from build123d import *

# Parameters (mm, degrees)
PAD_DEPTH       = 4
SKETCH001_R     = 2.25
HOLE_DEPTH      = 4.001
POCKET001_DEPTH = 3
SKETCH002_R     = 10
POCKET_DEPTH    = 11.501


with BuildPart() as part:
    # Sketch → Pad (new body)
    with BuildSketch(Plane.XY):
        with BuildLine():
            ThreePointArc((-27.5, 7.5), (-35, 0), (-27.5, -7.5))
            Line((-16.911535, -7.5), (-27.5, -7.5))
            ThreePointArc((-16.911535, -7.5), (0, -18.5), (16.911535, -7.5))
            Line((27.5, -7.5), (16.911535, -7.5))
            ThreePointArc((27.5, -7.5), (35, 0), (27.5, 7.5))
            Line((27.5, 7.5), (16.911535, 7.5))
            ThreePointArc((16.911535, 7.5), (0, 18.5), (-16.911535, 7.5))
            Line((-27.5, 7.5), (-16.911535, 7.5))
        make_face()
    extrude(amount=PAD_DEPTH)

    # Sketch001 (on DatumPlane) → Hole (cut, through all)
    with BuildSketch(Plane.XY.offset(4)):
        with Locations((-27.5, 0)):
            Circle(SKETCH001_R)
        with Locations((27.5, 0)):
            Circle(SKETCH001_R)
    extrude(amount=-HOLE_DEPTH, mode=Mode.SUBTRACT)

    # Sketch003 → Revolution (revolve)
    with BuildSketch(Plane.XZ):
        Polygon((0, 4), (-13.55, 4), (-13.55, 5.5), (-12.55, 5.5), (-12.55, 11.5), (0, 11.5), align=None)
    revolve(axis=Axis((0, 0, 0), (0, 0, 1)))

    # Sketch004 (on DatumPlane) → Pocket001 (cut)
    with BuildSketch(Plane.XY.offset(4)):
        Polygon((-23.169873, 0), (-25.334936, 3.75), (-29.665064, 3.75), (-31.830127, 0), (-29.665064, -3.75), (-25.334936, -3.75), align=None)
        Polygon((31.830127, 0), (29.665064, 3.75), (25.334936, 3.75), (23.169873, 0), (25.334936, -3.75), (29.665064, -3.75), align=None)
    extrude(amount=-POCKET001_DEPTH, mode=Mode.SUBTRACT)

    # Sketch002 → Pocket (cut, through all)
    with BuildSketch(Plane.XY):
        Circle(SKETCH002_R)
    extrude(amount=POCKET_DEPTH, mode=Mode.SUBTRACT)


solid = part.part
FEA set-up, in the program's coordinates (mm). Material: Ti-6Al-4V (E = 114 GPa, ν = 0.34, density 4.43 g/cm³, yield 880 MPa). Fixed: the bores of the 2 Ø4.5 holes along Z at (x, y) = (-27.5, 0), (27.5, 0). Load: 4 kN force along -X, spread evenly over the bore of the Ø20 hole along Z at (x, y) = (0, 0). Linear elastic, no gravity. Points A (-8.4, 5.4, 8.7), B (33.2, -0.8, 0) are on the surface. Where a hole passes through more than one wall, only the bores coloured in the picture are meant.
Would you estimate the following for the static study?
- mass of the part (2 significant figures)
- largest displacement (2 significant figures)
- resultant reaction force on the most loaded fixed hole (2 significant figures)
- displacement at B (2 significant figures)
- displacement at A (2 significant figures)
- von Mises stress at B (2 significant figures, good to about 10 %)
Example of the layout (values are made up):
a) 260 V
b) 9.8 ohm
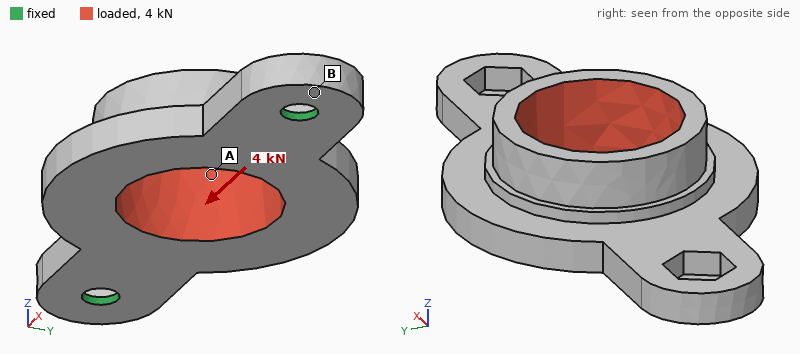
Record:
a) 27 g
b) 18 µm
c) 2.0 kN
d) 3.9 µm
e) 15 µm
f) 38 MPa
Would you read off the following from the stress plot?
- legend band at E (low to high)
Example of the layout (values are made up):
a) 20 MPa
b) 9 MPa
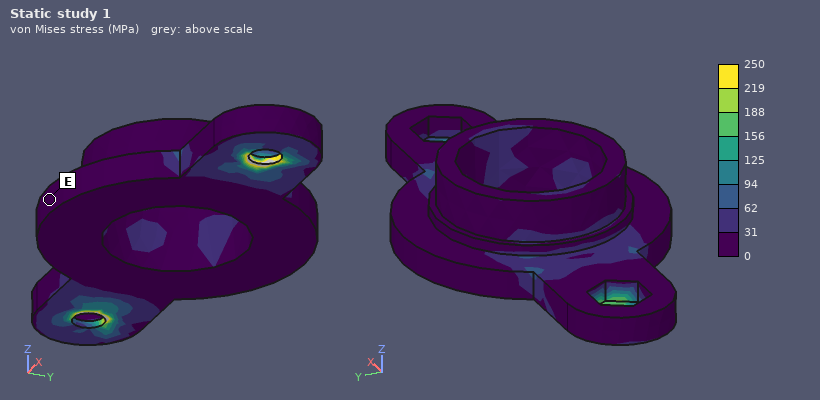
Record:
a) 0 to 31 MPa
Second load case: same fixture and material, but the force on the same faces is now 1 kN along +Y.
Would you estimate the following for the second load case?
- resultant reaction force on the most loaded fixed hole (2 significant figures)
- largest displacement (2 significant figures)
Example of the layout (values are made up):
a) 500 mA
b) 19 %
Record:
a) 500 N
b) 0.12 mm
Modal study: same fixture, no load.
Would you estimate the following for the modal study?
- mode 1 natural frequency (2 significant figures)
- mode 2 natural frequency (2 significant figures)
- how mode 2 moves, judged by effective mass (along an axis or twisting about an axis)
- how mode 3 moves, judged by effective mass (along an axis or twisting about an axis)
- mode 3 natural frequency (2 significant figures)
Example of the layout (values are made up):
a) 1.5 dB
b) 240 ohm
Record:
a) 2900 Hz
b) 4500 Hz
c) along Z
d) twisting about Y
e) 11 kHz
